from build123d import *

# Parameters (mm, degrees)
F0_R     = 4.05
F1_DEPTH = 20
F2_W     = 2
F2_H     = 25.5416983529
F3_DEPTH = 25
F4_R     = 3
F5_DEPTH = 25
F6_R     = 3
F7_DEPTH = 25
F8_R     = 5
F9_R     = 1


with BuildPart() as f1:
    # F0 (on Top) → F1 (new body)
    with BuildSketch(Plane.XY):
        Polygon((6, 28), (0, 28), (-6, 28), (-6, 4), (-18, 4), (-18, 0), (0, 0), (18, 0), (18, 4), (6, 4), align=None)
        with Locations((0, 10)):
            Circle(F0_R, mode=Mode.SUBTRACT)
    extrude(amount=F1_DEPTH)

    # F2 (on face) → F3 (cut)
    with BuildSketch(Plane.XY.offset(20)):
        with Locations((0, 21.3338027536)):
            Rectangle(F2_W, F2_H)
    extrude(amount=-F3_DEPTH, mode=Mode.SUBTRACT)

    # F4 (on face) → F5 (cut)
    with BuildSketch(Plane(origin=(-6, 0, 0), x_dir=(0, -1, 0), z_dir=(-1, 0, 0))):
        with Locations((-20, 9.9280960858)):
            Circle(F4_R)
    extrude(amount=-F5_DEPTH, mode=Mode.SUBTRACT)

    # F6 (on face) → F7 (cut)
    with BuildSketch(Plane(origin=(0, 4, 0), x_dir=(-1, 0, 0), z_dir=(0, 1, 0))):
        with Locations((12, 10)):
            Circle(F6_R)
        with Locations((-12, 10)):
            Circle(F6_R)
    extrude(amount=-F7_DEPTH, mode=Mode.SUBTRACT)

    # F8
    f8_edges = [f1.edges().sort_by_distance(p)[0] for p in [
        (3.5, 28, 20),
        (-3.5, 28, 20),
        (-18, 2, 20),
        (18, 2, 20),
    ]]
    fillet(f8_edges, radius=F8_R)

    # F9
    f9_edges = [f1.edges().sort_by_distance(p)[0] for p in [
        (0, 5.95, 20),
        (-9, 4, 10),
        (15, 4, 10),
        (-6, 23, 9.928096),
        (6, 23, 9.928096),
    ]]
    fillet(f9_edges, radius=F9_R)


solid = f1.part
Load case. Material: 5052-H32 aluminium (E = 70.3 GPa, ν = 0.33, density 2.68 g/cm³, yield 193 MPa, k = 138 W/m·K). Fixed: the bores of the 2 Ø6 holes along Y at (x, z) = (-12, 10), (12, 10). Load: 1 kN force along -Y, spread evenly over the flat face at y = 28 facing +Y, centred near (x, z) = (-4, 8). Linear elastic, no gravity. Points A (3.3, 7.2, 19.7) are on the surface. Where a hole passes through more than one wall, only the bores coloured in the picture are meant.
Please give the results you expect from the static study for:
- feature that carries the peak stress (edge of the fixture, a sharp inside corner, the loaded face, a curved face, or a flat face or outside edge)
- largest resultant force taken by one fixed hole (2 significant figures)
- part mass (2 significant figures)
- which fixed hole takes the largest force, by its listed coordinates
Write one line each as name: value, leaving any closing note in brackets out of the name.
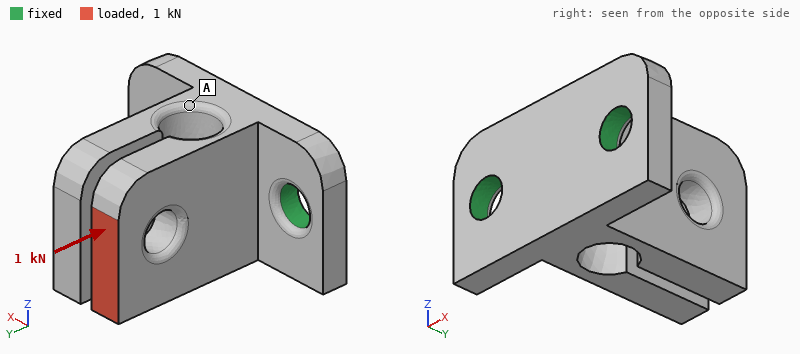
feature that carries the peak stress: a curved face
largest resultant force taken by one fixed hole: 750 N
part mass: 17 g
which fixed hole takes the largest force, by its listed coordinates: (-12, 10)
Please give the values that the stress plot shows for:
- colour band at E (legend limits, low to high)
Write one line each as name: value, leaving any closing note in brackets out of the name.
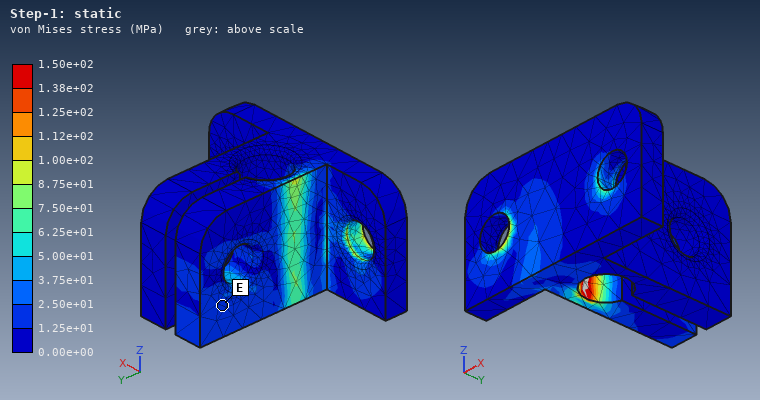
colour band at E: 1.25e+01 to 2.50e+01 MPa
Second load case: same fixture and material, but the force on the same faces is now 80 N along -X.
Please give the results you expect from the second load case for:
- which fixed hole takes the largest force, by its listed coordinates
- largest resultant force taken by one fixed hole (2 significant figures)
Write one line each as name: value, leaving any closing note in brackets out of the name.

which fixed hole takes the largest force, by its listed coordinates: (12, 10)
largest resultant force taken by one fixed hole: 150 N
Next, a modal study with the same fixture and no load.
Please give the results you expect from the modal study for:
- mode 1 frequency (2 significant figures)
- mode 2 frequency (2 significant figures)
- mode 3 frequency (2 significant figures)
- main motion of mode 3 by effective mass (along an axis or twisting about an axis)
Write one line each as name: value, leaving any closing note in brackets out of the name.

mode 1 frequency: 3000 Hz
mode 2 frequency: 3000 Hz
mode 3 frequency: 5500 Hz
main motion of mode 3 by effective mass: along Z
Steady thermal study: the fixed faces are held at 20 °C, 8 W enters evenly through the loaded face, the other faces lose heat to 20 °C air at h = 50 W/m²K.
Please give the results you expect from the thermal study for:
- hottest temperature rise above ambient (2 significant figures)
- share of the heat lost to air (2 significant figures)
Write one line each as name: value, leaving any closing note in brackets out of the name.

hottest temperature rise above ambient: 24 K
share of the heat lost to air: 13 %
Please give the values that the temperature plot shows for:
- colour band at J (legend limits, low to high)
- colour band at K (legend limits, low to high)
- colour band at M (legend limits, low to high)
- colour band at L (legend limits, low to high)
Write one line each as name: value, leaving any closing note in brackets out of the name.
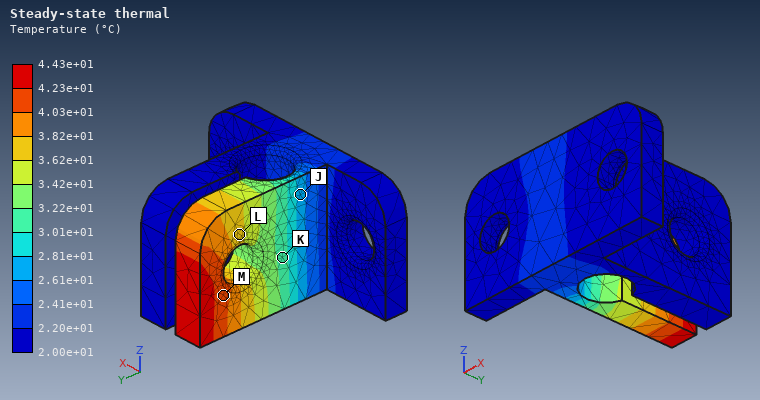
colour band at J: 2.61e+01 to 2.81e+01 °C
colour band at K: 3.01e+01 to 3.22e+01 °C
colour band at M: 4.03e+01 to 4.23e+01 °C
colour band at L: 3.62e+01 to 3.82e+01 °C
